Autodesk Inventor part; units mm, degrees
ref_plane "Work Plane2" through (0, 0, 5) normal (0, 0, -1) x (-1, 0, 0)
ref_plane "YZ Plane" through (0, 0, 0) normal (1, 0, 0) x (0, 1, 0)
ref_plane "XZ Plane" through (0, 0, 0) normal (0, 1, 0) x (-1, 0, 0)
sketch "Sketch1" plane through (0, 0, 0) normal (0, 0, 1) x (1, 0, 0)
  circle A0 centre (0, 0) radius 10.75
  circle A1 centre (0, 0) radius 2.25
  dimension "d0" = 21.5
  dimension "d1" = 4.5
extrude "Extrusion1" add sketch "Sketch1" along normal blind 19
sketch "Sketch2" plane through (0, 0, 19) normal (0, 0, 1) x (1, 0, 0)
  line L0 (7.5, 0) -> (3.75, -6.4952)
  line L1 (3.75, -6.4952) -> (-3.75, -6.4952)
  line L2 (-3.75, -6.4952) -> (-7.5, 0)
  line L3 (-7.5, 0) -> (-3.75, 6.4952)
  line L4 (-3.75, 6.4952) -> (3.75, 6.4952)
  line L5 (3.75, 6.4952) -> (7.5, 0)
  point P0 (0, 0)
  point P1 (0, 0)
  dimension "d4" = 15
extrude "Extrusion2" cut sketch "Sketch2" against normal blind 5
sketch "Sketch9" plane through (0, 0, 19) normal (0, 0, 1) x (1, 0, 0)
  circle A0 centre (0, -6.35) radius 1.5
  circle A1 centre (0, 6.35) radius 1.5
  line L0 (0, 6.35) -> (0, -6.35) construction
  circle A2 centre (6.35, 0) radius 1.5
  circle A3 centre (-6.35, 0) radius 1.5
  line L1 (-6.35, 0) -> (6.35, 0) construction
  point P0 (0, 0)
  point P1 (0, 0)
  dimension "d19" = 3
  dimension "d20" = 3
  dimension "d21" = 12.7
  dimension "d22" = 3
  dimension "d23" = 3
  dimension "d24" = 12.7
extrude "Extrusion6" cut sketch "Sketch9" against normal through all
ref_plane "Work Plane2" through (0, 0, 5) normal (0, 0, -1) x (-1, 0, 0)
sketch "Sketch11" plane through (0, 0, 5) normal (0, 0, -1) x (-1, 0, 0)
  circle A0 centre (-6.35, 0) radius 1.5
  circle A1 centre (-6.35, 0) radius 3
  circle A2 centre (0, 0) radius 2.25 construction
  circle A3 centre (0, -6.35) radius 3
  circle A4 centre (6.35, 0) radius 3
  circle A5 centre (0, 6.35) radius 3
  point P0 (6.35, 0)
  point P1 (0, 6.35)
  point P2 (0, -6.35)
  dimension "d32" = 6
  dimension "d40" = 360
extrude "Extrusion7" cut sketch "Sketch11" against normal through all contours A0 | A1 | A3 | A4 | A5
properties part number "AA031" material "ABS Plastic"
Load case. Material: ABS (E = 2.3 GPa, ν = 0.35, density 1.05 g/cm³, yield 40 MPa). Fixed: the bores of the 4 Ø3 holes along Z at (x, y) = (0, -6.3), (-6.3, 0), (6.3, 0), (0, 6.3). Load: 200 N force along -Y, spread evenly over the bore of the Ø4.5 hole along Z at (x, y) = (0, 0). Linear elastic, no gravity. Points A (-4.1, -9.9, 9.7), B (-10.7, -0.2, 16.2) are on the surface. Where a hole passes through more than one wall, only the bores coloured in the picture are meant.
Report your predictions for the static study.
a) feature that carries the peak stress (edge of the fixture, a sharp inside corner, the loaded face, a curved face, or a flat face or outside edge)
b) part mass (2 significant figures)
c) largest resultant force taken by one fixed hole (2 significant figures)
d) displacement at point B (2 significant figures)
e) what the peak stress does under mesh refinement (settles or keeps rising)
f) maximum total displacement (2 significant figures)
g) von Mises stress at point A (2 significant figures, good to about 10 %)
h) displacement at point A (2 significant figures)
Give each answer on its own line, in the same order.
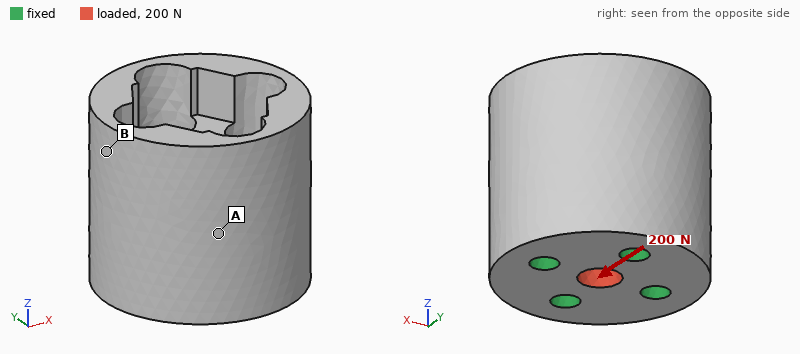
edge of the fixture
4.8 g
72 N
12 µm
keeps rising
20 µm
0.89 MPa
10 µm
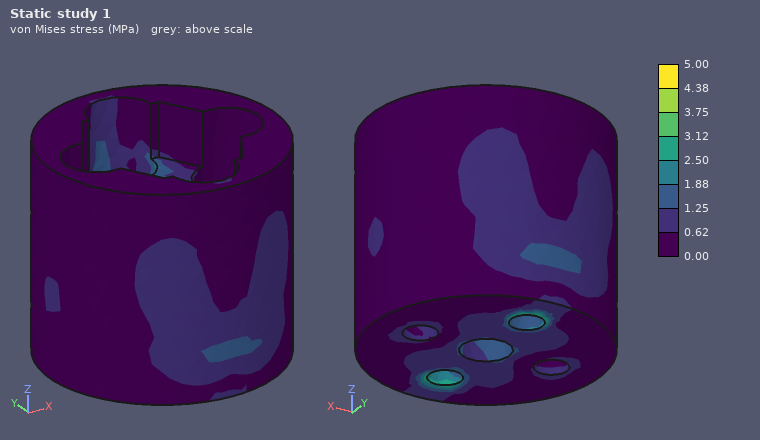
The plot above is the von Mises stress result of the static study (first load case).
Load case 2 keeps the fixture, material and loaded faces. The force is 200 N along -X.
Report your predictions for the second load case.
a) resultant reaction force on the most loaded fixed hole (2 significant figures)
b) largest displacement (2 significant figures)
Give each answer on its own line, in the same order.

72 N
20 µm
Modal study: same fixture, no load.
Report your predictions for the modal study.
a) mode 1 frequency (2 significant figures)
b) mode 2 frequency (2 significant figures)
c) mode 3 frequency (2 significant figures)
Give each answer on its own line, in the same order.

7700 Hz
7700 Hz
10 kHz
